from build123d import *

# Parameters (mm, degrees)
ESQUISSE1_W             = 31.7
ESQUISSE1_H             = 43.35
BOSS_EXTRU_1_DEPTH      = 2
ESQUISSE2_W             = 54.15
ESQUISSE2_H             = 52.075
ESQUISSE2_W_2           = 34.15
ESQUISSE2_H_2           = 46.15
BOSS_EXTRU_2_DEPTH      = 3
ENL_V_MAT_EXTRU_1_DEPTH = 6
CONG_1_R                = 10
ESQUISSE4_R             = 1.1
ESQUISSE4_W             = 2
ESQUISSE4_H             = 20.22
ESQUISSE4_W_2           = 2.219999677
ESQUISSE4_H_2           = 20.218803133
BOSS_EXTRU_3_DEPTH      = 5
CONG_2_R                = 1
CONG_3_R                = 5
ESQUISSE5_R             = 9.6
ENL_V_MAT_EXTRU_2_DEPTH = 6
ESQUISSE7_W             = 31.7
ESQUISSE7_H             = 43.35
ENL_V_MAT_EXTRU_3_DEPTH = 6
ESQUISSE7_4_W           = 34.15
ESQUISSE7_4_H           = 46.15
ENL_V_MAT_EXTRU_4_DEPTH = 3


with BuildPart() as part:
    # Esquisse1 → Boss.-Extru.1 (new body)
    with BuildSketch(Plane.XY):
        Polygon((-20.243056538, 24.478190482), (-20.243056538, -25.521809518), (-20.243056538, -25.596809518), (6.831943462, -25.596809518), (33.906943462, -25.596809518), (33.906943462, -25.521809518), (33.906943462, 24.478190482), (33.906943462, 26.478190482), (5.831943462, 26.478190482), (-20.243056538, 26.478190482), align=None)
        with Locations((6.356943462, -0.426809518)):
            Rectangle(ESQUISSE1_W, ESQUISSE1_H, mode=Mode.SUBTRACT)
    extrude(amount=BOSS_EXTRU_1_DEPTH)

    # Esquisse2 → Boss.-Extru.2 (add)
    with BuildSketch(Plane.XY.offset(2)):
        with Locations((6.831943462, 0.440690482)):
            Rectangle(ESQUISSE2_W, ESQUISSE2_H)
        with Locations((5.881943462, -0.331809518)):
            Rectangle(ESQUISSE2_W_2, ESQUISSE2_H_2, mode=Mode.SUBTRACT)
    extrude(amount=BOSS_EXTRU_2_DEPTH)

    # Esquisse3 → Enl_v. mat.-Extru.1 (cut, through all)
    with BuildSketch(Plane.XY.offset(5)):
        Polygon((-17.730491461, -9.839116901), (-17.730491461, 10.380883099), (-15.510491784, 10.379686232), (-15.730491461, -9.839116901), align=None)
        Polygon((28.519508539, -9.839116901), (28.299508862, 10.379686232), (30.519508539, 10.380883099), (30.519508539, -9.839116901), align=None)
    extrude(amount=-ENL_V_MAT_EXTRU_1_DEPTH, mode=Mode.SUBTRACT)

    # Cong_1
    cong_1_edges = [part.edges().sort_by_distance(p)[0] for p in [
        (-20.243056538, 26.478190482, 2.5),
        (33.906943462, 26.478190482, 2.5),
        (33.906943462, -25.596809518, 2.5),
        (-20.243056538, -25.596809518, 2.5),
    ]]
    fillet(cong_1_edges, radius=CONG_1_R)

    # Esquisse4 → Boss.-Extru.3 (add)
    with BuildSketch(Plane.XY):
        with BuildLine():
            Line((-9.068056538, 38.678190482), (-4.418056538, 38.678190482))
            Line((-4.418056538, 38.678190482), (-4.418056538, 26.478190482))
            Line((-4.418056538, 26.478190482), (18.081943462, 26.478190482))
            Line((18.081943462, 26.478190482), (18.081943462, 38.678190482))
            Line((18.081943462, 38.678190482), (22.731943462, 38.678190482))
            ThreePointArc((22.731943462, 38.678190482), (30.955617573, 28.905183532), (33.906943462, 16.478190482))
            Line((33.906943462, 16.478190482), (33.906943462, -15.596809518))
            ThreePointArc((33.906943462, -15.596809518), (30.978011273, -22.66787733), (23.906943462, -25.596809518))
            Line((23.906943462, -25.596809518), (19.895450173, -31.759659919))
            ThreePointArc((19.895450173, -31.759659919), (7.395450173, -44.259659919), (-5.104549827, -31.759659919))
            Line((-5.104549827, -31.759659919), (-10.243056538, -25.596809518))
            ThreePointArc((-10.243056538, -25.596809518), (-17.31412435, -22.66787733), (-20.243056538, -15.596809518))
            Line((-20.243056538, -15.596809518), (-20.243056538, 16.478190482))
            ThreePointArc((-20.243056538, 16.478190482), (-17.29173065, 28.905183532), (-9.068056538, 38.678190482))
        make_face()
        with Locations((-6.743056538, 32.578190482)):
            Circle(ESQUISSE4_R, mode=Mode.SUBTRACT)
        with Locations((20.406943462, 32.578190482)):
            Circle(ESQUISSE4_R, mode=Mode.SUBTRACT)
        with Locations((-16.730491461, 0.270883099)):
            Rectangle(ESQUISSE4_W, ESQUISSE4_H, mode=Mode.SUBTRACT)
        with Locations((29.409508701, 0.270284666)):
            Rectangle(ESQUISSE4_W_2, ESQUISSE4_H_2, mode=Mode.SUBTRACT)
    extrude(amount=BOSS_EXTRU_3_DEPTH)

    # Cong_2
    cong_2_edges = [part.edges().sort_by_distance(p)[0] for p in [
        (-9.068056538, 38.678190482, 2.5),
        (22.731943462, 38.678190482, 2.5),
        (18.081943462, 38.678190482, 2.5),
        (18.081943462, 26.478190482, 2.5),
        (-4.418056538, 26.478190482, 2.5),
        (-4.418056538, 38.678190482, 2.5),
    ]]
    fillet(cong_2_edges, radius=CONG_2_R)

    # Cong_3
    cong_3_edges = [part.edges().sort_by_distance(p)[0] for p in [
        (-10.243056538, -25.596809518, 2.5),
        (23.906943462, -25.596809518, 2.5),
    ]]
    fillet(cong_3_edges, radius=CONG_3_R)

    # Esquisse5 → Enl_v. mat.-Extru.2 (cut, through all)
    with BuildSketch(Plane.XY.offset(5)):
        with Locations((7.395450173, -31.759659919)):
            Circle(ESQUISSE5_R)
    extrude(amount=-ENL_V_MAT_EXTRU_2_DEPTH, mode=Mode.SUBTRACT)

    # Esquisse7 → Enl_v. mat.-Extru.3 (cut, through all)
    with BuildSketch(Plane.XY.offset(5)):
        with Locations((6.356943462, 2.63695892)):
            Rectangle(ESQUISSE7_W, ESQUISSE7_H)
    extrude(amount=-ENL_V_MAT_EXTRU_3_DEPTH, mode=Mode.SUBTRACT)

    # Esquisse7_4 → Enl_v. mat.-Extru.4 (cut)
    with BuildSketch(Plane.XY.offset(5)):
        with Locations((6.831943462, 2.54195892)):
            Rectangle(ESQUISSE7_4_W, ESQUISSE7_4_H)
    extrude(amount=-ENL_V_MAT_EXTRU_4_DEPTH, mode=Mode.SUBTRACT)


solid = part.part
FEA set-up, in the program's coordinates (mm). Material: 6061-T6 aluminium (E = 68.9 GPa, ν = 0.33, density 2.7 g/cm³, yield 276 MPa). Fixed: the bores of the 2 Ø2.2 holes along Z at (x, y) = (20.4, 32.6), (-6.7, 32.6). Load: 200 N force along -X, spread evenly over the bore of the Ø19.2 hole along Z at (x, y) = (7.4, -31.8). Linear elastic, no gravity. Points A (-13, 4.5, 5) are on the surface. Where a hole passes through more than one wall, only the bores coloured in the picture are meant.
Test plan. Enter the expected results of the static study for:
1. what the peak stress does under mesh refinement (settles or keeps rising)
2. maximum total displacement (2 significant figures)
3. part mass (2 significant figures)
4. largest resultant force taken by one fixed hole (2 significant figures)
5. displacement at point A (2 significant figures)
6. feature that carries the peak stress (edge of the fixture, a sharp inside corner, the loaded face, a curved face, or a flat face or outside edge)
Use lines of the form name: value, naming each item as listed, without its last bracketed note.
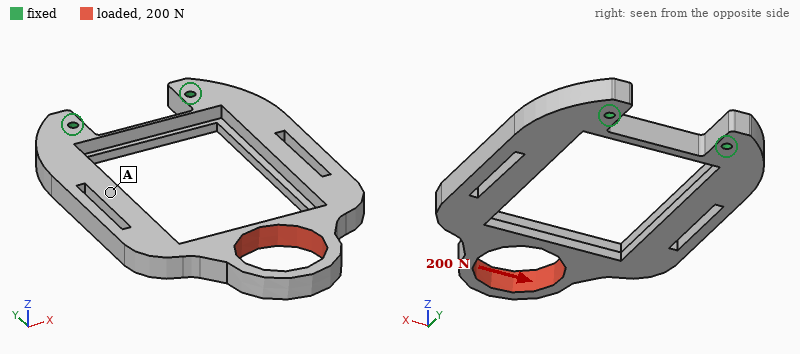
what the peak stress does under mesh refinement: keeps rising
maximum total displacement: 0.26 mm
part mass: 21 g
largest resultant force taken by one fixed hole: 200 N
displacement at point A: 0.11 mm
feature that carries the peak stress: edge of the fixture
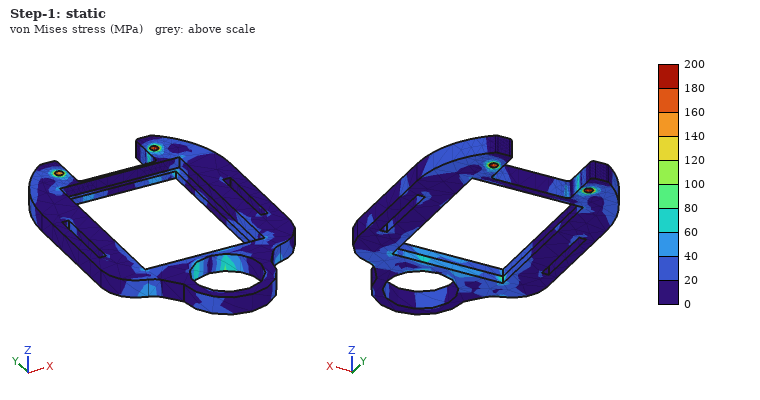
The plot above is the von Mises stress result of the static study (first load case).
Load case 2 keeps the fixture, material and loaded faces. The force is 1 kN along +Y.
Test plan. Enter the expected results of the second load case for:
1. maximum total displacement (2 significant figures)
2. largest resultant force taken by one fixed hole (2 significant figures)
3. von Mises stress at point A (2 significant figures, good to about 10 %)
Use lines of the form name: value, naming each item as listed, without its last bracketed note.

maximum total displacement: 84 µm
largest resultant force taken by one fixed hole: 540 N
von Mises stress at point A: 24 MPa
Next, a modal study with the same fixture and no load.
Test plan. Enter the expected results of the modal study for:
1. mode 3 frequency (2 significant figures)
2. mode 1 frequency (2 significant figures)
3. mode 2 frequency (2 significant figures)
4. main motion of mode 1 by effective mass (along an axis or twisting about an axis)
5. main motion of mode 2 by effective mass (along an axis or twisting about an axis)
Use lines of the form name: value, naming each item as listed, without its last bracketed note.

mode 3 frequency: 1800 Hz
mode 1 frequency: 720 Hz
mode 2 frequency: 1500 Hz
main motion of mode 1 by effective mass: along Z
main motion of mode 2 by effective mass: along X
